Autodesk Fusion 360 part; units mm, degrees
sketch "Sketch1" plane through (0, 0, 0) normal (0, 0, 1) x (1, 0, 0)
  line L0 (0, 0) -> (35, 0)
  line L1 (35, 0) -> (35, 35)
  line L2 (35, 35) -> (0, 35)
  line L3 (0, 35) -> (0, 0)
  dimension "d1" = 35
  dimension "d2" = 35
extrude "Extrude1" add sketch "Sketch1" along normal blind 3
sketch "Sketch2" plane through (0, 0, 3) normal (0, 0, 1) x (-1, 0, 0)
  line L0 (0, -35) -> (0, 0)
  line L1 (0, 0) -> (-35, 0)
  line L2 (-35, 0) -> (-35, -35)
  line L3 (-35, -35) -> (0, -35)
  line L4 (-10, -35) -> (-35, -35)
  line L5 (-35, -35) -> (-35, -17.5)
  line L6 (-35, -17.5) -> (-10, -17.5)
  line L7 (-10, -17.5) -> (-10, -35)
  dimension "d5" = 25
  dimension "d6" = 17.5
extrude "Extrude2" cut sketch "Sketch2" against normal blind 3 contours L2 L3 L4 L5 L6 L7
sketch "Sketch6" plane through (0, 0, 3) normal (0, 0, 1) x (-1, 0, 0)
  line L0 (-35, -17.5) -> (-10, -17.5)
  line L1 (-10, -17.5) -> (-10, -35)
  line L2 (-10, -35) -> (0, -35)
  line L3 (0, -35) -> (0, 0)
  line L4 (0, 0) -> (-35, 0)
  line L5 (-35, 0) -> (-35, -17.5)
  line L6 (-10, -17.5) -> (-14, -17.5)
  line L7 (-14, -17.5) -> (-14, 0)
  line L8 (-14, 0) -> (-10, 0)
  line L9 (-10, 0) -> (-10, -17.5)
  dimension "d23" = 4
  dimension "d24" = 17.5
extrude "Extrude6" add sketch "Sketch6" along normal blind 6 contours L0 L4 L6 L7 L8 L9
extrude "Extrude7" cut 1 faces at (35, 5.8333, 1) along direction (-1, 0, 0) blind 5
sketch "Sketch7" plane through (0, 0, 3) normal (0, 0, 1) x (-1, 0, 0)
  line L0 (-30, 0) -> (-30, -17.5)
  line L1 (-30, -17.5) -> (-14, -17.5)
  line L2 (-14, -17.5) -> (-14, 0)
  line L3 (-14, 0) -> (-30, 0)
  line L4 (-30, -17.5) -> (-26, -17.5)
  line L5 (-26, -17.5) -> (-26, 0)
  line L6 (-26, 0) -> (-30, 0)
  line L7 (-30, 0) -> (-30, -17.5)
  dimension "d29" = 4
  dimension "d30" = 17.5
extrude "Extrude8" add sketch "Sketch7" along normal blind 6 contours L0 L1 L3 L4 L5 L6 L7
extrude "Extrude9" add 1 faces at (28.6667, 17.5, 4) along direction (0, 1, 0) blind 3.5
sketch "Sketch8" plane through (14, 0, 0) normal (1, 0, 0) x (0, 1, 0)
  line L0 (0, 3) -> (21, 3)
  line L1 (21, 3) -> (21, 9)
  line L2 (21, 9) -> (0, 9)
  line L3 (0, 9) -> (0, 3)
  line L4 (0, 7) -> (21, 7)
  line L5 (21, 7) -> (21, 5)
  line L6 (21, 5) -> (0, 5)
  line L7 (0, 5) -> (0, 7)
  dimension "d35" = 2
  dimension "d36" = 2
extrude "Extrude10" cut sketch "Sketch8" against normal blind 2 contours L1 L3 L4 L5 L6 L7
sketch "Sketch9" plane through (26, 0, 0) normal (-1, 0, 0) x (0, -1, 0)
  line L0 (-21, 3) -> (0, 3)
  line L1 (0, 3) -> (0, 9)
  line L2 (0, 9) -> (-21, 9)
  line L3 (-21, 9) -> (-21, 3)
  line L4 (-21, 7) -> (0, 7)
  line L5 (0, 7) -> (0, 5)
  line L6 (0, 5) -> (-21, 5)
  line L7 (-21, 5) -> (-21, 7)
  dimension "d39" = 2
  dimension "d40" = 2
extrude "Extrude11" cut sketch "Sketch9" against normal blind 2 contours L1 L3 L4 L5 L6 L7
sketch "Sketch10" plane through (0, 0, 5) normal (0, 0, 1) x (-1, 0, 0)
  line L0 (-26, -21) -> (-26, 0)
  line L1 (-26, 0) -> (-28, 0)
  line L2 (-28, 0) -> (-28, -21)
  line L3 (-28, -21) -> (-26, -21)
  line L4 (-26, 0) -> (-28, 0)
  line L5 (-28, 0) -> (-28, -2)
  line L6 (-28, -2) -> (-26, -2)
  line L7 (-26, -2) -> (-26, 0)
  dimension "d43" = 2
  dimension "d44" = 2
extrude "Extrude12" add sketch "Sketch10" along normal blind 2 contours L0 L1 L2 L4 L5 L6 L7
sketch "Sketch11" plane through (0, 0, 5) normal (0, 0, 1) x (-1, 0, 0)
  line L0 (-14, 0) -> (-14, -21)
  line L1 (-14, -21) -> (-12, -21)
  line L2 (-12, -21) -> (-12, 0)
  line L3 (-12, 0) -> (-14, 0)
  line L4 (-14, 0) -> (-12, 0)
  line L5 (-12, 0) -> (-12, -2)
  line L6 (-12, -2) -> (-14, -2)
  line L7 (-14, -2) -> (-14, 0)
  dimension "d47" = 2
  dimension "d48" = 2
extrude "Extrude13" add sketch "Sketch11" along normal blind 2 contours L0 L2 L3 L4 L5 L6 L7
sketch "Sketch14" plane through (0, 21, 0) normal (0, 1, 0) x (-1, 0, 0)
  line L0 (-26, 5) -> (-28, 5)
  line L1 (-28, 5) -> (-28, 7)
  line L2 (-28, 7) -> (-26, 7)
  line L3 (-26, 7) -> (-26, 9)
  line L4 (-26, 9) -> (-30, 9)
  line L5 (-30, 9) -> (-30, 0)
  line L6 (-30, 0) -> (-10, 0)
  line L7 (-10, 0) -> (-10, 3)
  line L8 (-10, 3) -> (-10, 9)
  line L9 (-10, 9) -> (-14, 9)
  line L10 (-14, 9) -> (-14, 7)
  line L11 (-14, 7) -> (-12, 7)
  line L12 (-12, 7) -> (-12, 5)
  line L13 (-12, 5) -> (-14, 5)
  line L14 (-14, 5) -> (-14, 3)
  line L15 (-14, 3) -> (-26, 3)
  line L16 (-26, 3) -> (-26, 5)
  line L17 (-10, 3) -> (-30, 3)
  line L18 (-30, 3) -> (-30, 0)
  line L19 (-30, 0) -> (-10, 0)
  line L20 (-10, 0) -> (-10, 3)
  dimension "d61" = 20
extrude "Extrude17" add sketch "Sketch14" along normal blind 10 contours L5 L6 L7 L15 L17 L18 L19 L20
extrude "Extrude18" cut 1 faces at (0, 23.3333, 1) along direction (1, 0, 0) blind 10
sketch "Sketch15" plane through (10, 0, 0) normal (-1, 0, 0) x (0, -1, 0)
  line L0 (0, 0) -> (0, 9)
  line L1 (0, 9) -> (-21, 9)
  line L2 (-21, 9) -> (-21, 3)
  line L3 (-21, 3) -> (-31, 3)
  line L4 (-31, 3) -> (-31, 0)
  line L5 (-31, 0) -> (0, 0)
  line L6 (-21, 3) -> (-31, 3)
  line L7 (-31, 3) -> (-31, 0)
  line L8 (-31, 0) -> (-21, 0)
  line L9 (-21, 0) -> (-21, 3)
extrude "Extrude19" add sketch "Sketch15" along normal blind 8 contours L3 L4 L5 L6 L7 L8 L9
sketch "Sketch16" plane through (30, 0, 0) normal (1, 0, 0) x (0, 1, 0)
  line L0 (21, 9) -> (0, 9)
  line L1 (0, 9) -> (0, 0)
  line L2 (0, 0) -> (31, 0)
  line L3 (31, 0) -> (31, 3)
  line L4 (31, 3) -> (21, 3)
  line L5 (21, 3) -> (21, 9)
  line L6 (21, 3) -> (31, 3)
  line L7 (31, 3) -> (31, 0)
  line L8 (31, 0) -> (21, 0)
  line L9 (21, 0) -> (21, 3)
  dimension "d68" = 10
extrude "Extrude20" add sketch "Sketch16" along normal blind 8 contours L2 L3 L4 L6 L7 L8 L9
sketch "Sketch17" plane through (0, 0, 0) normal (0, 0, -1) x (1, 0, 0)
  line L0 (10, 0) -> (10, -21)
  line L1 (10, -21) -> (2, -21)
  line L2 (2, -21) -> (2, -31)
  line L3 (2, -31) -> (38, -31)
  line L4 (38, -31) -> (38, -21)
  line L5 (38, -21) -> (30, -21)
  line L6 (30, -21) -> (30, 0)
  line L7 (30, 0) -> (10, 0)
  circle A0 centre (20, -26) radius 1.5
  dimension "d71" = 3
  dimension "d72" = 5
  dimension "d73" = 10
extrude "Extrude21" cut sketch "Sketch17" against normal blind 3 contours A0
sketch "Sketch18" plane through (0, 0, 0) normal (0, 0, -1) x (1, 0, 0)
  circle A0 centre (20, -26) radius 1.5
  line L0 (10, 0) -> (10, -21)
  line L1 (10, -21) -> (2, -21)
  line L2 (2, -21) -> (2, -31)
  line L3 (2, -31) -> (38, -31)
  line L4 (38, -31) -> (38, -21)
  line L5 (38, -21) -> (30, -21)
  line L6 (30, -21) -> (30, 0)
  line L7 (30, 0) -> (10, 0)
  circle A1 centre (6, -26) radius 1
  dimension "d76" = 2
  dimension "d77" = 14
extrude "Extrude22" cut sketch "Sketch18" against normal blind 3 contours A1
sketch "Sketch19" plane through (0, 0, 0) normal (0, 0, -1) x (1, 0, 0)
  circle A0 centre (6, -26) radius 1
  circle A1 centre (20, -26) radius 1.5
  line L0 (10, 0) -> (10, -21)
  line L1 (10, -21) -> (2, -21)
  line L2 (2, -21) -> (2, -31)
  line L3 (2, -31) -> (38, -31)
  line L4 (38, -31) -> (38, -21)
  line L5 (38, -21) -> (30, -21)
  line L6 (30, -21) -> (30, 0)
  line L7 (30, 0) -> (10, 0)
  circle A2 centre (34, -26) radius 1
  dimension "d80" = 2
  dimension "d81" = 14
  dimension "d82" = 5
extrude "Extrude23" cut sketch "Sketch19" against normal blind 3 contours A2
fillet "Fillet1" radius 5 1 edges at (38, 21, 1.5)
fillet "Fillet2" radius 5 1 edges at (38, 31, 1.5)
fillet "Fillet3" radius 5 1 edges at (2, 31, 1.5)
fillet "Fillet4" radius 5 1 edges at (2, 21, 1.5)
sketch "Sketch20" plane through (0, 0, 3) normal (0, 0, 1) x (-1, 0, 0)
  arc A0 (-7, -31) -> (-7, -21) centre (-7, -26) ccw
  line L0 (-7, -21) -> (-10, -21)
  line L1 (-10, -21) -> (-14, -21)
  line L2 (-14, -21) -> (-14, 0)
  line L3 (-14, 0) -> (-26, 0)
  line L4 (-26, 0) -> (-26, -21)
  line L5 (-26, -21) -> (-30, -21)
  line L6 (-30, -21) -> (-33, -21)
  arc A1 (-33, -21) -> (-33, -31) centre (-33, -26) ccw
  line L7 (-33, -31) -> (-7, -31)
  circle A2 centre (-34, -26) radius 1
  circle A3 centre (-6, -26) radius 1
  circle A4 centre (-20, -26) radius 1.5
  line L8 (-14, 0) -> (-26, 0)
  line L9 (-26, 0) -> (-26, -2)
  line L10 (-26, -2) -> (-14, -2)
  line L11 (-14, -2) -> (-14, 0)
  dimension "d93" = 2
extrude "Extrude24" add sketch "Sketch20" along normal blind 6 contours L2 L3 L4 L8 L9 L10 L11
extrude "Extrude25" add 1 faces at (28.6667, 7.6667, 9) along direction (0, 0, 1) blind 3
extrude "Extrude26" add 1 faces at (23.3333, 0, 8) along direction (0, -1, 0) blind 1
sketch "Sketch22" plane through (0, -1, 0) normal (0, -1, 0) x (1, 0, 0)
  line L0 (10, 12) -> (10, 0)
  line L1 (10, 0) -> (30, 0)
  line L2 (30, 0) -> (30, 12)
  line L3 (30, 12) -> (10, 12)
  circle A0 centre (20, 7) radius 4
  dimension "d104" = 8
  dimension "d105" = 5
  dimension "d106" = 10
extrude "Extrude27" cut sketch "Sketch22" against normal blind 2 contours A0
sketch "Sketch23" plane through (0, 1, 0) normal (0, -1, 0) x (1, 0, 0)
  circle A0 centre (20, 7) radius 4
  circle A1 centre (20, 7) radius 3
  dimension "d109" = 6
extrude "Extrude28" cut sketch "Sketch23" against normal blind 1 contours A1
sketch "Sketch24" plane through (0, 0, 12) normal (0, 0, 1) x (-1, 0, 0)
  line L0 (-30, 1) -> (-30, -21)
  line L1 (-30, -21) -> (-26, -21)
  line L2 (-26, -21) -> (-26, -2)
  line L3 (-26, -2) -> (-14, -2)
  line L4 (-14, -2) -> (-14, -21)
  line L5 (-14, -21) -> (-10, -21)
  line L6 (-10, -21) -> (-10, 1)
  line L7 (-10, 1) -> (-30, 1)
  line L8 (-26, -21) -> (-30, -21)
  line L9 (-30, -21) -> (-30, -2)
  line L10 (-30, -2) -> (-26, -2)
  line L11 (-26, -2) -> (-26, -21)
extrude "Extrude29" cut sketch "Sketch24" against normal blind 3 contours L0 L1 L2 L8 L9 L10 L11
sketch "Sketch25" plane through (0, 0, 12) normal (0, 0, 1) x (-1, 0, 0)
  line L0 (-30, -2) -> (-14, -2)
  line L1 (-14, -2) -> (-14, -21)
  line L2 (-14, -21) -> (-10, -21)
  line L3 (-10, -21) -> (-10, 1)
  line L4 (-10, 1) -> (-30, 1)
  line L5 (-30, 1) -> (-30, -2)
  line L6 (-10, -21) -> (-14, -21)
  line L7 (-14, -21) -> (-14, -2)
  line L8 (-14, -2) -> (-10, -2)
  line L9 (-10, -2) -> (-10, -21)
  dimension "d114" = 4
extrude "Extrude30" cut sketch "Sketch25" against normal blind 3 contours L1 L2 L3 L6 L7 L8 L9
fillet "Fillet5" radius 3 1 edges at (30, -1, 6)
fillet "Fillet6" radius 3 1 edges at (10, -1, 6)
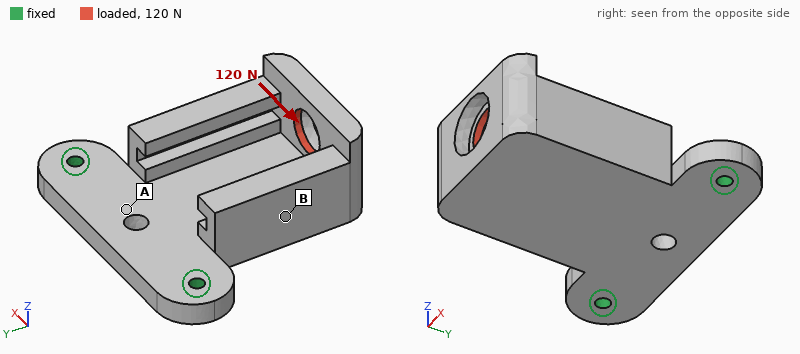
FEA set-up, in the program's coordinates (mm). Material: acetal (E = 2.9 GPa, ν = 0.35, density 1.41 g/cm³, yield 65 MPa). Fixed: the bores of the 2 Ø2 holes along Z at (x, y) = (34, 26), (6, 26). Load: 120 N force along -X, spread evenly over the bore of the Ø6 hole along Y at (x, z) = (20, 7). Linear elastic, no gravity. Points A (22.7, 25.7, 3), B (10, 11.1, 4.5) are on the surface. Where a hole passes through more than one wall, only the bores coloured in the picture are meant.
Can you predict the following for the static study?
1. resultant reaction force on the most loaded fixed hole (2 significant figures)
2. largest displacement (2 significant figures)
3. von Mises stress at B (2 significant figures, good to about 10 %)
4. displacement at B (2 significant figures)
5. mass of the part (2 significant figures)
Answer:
130 N
0.56 mm
8.7 MPa
0.22 mm
4.8 g
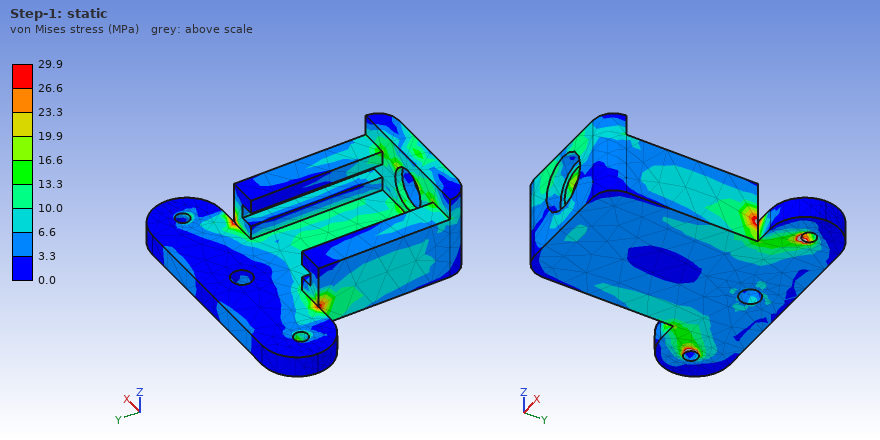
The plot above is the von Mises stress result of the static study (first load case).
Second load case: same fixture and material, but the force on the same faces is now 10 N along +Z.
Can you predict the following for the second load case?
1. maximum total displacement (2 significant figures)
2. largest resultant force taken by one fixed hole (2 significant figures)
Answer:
0.51 mm
5.1 N
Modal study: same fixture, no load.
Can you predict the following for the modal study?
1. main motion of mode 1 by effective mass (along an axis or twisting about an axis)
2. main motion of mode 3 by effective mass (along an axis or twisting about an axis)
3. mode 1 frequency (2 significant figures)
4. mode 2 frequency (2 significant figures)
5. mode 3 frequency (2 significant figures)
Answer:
along Z
along X
560 Hz
2000 Hz
3400 Hz
